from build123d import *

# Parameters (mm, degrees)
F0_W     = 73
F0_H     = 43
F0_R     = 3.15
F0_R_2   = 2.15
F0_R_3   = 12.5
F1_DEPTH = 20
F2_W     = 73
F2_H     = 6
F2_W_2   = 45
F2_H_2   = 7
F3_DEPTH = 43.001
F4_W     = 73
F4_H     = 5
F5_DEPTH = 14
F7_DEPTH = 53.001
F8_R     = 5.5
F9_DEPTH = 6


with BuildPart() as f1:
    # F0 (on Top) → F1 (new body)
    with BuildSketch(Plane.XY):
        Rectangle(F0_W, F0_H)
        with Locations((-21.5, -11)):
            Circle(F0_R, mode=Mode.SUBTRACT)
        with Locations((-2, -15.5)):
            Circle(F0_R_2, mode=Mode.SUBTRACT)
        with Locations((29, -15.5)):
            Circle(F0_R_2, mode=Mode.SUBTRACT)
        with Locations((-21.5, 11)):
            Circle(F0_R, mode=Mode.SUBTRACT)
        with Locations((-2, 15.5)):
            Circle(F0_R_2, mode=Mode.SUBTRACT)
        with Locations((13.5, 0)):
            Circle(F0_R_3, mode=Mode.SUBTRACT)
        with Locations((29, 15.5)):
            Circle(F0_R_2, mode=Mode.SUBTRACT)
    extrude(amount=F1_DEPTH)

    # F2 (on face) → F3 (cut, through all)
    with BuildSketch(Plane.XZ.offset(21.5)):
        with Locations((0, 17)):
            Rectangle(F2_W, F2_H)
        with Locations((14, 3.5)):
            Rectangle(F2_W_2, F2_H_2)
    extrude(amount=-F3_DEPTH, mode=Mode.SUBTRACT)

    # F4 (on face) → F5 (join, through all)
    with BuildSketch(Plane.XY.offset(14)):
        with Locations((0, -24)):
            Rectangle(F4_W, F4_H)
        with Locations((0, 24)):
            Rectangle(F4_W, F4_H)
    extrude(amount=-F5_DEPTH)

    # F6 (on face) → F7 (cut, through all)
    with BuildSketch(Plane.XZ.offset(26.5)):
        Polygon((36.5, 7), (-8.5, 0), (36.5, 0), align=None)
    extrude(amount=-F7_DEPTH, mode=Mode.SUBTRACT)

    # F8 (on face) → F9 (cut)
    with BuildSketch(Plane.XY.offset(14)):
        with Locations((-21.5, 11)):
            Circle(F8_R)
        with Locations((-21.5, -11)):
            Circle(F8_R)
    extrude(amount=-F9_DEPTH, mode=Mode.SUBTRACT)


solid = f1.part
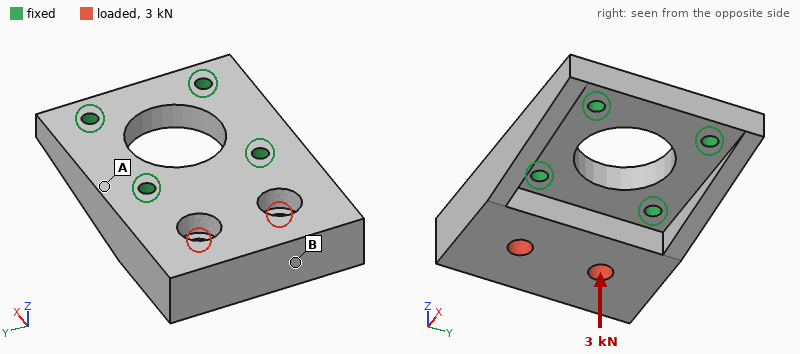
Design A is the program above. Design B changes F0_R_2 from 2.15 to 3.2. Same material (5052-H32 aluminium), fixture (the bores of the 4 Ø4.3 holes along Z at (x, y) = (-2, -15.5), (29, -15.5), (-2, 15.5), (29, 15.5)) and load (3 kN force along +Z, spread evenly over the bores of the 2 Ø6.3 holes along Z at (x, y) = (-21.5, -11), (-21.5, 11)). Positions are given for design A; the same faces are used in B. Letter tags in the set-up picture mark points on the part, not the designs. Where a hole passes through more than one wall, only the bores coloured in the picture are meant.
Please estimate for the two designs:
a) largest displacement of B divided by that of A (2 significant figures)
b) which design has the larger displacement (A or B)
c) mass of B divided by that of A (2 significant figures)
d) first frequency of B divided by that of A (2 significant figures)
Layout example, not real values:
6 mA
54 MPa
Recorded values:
0.81
A
0.99
1.1
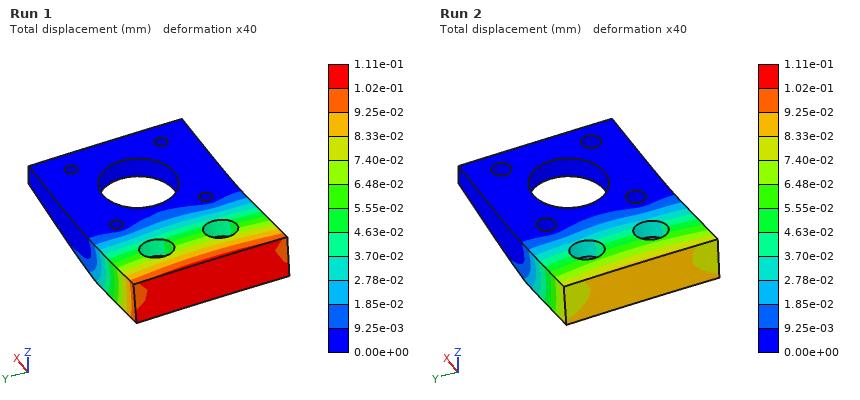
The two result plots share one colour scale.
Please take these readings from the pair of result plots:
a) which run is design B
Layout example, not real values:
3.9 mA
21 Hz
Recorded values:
Run 2
